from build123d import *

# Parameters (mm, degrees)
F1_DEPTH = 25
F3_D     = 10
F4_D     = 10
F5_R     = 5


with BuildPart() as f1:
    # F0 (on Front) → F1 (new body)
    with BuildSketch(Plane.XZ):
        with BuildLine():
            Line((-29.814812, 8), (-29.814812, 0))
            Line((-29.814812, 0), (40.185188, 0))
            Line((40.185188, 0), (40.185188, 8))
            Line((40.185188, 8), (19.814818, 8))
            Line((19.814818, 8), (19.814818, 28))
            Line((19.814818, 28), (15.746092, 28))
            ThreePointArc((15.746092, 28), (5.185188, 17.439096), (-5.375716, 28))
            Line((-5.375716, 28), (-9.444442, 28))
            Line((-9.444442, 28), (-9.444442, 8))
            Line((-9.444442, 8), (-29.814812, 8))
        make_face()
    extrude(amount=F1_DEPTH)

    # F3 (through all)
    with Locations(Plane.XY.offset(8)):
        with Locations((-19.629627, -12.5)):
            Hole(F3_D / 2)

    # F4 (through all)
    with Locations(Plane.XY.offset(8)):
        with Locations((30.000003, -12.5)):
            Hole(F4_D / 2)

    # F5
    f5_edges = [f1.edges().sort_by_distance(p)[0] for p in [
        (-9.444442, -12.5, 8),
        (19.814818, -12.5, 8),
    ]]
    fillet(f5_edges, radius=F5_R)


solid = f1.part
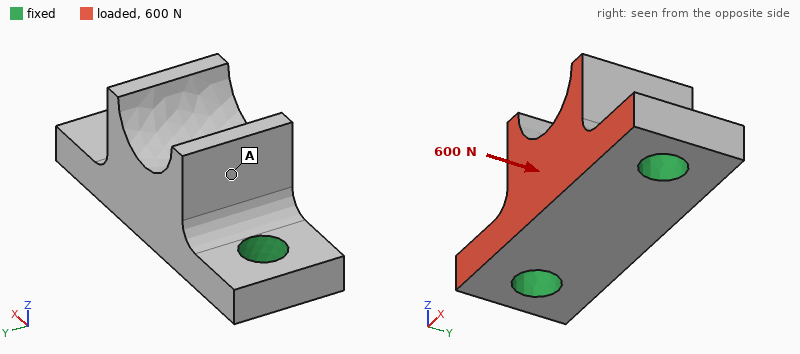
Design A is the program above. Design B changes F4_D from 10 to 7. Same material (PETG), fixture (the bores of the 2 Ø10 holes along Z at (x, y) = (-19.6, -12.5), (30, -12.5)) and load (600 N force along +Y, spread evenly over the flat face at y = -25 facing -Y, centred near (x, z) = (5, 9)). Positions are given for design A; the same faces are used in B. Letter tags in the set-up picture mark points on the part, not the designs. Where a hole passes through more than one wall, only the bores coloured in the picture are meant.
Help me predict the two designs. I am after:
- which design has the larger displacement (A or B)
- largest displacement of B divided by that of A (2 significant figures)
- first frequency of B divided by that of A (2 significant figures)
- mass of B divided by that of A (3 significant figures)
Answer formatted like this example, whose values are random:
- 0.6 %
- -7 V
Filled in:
- B
- 1.2
- 0.93
- 1.01
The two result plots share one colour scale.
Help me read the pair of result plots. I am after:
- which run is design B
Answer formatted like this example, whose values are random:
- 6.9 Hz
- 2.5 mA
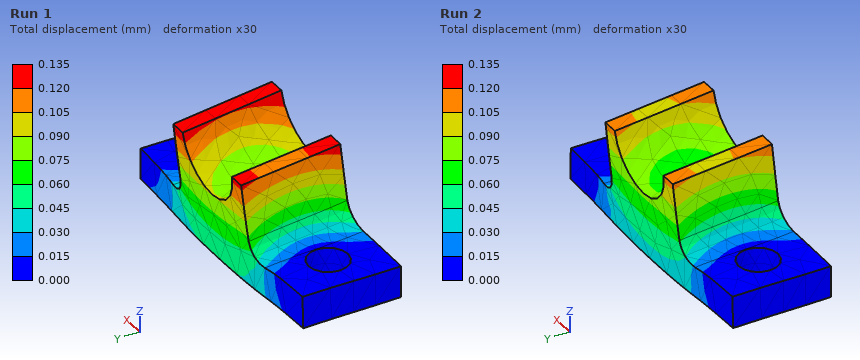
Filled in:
- Run 1
